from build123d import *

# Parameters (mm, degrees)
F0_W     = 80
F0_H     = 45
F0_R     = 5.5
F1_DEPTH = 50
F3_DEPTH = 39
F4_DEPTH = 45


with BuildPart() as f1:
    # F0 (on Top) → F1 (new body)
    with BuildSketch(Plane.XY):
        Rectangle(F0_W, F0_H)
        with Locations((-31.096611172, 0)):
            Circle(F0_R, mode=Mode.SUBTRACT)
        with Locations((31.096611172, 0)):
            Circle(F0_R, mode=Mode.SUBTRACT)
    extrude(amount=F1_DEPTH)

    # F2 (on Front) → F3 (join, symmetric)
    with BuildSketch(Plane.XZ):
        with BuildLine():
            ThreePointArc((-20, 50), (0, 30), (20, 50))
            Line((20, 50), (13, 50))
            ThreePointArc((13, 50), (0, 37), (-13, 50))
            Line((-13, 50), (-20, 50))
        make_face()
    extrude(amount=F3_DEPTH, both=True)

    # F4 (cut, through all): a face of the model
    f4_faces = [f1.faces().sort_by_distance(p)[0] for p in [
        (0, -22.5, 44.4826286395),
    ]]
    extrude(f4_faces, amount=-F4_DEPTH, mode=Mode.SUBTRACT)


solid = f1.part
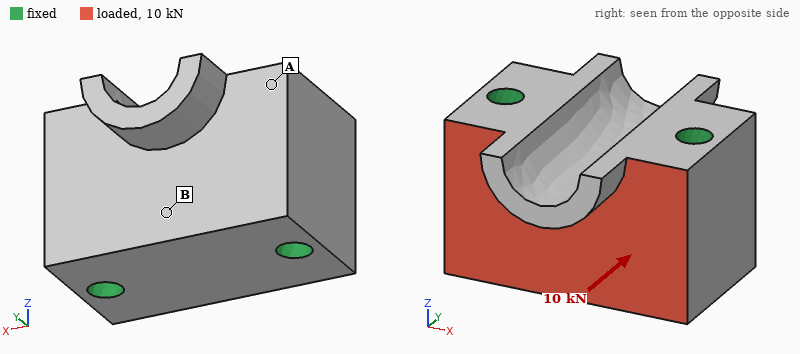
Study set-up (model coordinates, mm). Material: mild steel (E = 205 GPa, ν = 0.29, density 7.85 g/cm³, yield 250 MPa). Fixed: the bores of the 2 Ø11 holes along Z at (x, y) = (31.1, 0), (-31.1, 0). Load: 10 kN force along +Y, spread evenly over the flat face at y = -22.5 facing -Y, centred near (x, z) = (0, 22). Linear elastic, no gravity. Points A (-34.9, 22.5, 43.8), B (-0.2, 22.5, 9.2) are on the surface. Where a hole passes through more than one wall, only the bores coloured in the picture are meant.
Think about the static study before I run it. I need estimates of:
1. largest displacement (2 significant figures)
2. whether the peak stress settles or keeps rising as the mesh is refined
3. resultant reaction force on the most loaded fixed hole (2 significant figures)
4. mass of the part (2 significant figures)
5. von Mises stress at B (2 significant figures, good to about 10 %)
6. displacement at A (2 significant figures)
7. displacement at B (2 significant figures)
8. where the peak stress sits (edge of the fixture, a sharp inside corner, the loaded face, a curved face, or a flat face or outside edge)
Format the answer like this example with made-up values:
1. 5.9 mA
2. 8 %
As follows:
1. 0.88 µm
2. keeps rising
3. 5.0 kN
4. 1.3 kg
5. 2.6 MPa
6. 0.16 µm
7. 0.45 µm
8. edge of the fixture
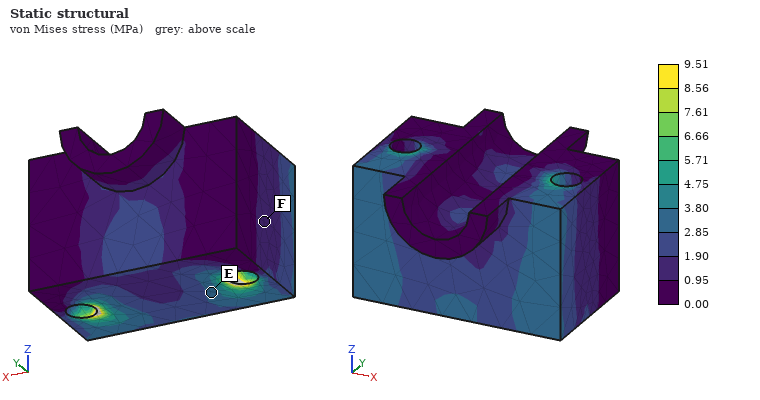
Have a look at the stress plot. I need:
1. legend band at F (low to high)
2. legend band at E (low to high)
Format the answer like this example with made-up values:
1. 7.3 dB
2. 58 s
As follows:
1. 0.95 to 1.90 MPa
2. 2.85 to 3.80 MPa
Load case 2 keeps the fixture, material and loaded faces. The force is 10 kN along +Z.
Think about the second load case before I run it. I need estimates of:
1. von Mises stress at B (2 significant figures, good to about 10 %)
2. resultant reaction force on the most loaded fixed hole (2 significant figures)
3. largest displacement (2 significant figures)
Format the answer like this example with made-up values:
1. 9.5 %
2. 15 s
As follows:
1. 1.9 MPa
2. 5.0 kN
3. 2.2 µm
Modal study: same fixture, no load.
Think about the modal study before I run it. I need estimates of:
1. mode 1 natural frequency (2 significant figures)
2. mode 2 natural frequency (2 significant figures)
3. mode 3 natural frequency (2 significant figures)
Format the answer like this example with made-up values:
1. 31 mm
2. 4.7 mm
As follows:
1. 17 kHz
2. 17 kHz
3. 17 kHz
